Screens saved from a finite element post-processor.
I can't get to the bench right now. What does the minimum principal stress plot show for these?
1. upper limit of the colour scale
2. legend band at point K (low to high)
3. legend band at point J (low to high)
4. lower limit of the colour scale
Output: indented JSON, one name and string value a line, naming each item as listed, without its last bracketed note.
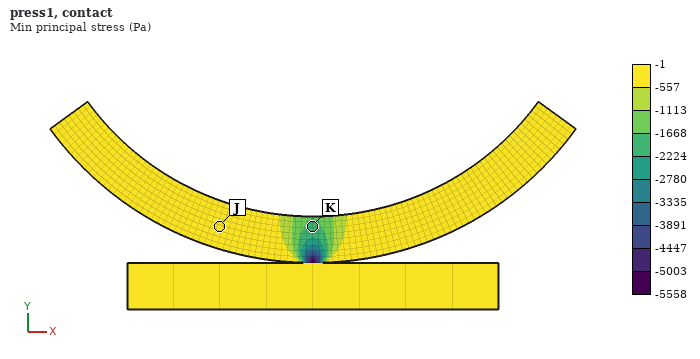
{
  "upper limit of the colour scale": "-1 Pa",
  "legend band at point K": "-2224 to -1668 Pa",
  "legend band at point J": "-557 to -1 Pa",
  "lower limit of the colour scale": "-5558 Pa"
}
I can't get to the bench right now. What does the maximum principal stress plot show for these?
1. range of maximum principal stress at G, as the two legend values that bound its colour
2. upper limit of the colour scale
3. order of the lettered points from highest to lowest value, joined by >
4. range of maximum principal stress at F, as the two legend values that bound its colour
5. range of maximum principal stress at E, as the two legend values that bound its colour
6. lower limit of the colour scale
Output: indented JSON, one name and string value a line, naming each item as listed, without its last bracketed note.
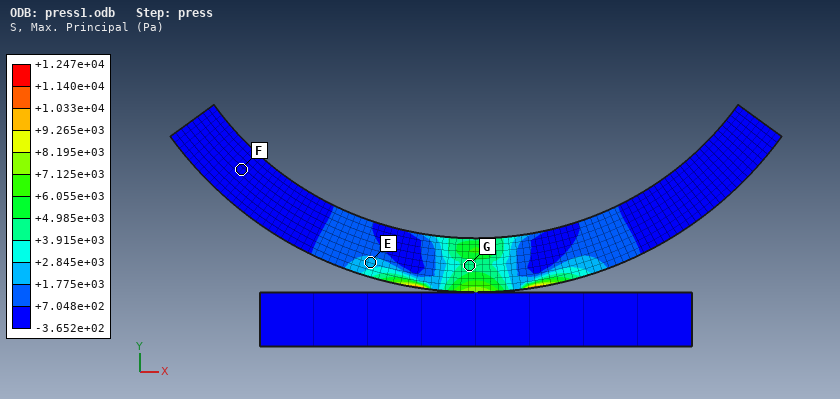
{
  "range of maximum principal stress at G, as the two legend values that bound its colour": "+3.915e+03 to +4.985e+03 Pa",
  "upper limit of the colour scale": "+1.247e+04 Pa",
  "order of the lettered points from highest to lowest value, joined by >": "G > E > F",
  "range of maximum principal stress at F, as the two legend values that bound its colour": "-3.652e+02 to +7.048e+02 Pa",
  "range of maximum principal stress at E, as the two legend values that bound its colour": "+1.775e+03 to +2.845e+03 Pa",
  "lower limit of the colour scale": "-3.652e+02 Pa"
}
